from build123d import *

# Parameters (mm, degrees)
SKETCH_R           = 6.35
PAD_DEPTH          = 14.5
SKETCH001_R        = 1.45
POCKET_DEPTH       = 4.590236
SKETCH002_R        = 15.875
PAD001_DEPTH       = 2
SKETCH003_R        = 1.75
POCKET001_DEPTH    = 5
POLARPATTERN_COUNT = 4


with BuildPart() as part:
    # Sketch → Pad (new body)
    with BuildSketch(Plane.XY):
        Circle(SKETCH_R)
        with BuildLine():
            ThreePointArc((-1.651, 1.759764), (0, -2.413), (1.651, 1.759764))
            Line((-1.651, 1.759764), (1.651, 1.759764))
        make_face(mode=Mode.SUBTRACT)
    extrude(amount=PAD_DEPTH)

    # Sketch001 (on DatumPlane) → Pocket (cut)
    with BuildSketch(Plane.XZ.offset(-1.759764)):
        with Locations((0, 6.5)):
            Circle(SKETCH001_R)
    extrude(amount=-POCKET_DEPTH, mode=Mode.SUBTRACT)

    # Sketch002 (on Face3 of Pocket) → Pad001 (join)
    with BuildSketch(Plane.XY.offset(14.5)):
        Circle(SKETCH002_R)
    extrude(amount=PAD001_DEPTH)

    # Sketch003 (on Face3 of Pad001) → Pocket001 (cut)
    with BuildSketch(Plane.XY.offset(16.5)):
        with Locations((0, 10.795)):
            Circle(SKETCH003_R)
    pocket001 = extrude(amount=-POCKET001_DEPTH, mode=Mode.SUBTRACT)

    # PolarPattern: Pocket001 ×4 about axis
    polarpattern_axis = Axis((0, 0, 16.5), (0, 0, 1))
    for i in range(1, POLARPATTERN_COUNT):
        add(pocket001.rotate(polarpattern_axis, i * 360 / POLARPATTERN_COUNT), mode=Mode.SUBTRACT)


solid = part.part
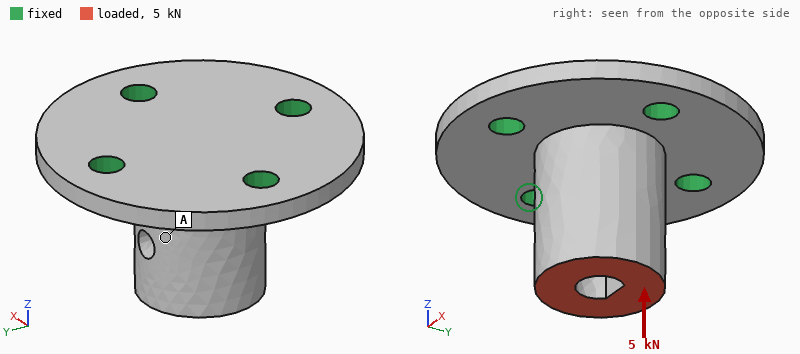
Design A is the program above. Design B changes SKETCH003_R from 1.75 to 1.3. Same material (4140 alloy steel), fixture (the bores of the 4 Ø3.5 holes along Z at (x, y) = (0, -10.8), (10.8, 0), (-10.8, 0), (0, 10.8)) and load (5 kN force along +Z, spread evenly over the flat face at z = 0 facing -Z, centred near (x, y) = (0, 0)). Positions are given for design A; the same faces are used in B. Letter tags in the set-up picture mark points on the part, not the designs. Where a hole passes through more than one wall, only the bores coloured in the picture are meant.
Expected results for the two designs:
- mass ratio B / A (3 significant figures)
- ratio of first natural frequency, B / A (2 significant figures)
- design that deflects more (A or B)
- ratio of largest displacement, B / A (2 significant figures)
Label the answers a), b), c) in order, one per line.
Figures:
a) 1.01
b) 0.92
c) B
d) 1.2
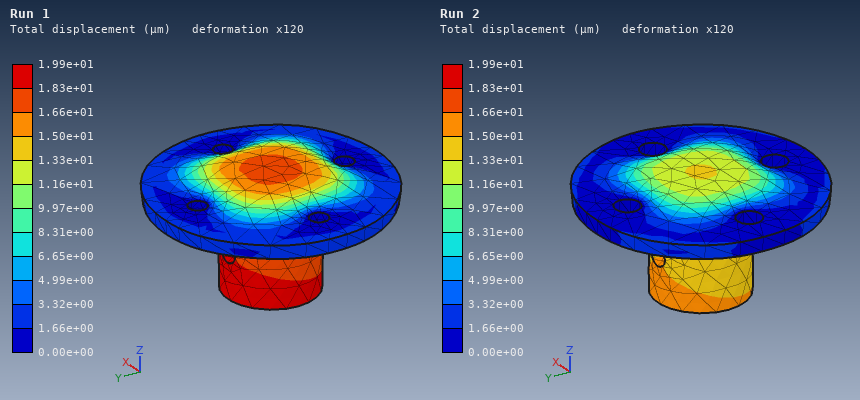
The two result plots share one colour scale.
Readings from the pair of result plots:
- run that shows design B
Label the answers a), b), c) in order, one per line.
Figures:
a) Run 1
